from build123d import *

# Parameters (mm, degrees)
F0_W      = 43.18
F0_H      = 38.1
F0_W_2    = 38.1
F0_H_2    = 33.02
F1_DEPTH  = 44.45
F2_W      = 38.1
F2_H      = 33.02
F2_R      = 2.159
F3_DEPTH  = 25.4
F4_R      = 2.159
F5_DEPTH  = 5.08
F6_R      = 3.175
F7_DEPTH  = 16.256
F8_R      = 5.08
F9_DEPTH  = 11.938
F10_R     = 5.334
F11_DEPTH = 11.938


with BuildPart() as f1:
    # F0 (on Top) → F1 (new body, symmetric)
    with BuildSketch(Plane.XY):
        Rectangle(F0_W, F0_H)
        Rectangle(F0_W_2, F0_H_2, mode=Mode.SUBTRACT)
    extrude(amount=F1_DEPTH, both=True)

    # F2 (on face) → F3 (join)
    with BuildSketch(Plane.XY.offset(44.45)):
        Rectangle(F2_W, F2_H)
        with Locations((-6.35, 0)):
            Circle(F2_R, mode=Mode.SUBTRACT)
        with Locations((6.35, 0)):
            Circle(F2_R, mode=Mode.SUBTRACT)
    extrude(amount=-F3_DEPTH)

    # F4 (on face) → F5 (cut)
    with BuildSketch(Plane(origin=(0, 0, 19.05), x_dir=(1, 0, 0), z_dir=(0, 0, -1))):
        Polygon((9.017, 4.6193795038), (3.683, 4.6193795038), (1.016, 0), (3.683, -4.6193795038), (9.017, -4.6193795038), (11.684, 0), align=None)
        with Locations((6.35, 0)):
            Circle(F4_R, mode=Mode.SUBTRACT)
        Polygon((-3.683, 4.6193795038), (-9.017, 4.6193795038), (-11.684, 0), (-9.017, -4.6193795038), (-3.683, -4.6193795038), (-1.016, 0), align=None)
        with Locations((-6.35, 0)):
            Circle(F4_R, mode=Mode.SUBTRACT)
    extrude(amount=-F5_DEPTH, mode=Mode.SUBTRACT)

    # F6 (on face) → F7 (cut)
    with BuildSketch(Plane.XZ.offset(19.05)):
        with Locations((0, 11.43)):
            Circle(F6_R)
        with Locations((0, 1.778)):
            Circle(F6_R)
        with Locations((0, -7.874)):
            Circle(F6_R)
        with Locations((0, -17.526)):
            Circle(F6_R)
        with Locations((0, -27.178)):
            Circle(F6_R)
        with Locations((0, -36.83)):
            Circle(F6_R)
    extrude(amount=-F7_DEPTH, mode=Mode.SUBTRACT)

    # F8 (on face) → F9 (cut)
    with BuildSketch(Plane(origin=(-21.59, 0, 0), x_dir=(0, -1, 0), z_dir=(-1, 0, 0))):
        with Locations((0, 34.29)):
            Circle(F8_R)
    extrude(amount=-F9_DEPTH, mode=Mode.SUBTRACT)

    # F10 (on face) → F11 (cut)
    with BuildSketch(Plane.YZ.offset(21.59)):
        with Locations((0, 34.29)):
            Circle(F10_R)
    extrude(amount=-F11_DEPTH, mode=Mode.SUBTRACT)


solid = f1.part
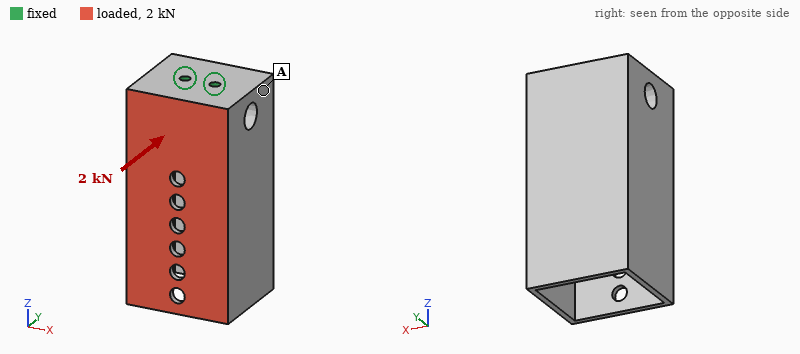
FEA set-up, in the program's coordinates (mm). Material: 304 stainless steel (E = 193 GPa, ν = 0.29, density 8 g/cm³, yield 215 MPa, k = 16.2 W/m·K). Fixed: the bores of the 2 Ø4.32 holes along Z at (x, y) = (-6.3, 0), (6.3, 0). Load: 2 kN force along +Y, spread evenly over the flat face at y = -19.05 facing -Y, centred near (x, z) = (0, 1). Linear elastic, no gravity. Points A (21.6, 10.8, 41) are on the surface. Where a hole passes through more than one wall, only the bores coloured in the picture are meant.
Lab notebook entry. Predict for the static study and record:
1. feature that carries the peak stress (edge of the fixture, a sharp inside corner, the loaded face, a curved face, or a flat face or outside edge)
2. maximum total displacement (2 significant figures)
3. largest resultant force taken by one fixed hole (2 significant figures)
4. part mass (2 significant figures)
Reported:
the loaded face
53 µm
1.0 kN
500 g
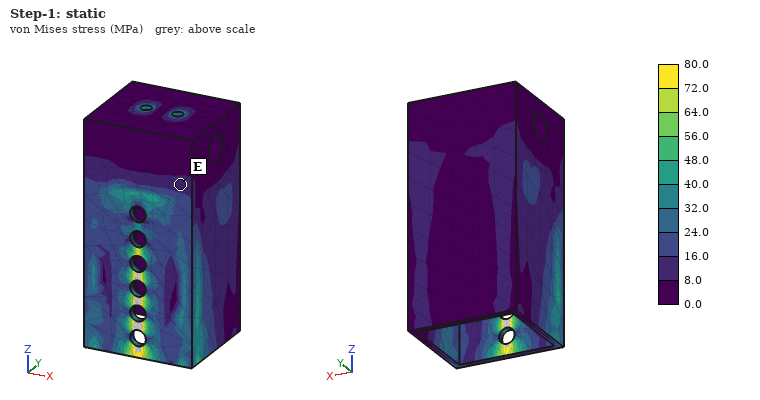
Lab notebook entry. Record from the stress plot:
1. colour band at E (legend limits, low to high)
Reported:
8.0 to 16.0 MPa
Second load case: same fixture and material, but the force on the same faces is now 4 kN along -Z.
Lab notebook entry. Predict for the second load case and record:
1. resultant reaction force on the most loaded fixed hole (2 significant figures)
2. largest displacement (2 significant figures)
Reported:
2.0 kN
24 µm
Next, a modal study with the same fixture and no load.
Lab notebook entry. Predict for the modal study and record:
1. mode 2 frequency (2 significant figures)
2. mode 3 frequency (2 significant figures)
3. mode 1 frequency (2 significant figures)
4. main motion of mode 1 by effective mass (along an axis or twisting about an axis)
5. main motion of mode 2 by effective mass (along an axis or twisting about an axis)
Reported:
3800 Hz
4200 Hz
3500 Hz
along Y
along X
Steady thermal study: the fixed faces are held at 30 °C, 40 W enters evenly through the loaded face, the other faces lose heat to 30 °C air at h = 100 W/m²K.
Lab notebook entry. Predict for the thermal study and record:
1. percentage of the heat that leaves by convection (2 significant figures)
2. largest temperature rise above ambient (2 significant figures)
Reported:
71 %
54 K
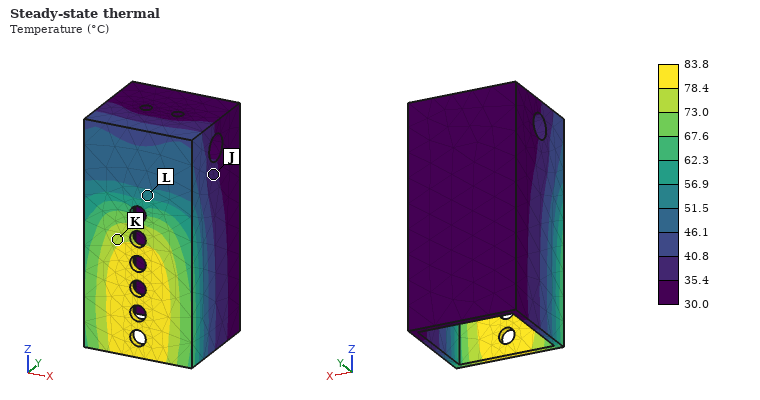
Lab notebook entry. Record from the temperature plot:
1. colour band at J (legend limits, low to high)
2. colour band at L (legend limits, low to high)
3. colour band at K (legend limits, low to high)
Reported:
35.4 to 40.8 °C
51.5 to 56.9 °C
73.0 to 78.4 °C
